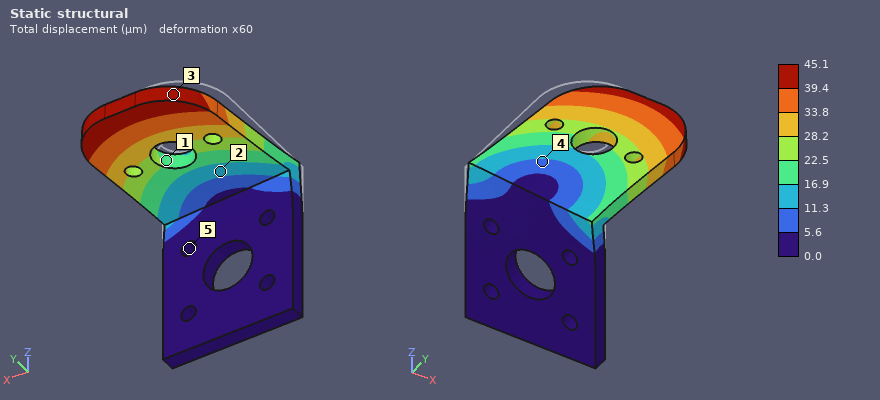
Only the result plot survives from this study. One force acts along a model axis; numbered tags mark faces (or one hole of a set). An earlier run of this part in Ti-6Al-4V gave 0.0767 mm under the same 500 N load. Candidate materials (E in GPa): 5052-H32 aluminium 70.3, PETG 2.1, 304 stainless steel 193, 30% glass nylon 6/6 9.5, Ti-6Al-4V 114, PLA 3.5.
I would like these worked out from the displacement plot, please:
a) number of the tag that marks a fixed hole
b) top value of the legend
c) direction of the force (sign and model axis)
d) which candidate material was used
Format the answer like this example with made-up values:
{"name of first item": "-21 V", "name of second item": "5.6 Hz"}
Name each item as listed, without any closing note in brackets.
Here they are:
{"number of the tag that marks a fixed hole": "5", "top value of the legend": "45.1 µm", "direction of the force": "+X", "which candidate material was used": "304 stainless steel"}
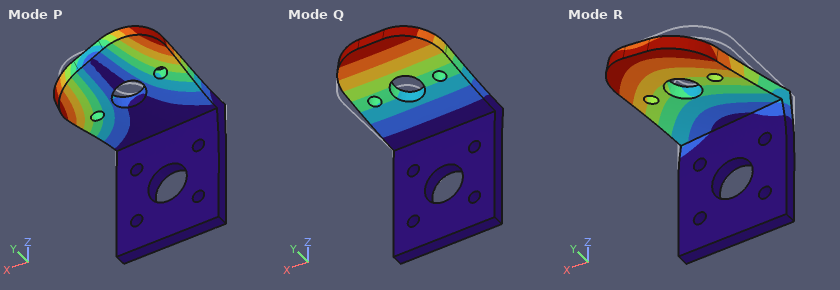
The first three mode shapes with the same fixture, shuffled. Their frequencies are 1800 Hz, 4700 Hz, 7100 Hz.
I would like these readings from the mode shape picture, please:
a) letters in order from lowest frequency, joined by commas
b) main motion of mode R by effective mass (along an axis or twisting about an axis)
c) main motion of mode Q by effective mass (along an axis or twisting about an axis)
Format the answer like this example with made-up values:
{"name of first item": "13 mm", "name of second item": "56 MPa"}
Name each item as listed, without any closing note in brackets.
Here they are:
{"letters in order from lowest frequency, joined by commas": "Q, R, P", "main motion of mode R by effective mass": "along X", "main motion of mode Q by effective mass": "along Z"}
